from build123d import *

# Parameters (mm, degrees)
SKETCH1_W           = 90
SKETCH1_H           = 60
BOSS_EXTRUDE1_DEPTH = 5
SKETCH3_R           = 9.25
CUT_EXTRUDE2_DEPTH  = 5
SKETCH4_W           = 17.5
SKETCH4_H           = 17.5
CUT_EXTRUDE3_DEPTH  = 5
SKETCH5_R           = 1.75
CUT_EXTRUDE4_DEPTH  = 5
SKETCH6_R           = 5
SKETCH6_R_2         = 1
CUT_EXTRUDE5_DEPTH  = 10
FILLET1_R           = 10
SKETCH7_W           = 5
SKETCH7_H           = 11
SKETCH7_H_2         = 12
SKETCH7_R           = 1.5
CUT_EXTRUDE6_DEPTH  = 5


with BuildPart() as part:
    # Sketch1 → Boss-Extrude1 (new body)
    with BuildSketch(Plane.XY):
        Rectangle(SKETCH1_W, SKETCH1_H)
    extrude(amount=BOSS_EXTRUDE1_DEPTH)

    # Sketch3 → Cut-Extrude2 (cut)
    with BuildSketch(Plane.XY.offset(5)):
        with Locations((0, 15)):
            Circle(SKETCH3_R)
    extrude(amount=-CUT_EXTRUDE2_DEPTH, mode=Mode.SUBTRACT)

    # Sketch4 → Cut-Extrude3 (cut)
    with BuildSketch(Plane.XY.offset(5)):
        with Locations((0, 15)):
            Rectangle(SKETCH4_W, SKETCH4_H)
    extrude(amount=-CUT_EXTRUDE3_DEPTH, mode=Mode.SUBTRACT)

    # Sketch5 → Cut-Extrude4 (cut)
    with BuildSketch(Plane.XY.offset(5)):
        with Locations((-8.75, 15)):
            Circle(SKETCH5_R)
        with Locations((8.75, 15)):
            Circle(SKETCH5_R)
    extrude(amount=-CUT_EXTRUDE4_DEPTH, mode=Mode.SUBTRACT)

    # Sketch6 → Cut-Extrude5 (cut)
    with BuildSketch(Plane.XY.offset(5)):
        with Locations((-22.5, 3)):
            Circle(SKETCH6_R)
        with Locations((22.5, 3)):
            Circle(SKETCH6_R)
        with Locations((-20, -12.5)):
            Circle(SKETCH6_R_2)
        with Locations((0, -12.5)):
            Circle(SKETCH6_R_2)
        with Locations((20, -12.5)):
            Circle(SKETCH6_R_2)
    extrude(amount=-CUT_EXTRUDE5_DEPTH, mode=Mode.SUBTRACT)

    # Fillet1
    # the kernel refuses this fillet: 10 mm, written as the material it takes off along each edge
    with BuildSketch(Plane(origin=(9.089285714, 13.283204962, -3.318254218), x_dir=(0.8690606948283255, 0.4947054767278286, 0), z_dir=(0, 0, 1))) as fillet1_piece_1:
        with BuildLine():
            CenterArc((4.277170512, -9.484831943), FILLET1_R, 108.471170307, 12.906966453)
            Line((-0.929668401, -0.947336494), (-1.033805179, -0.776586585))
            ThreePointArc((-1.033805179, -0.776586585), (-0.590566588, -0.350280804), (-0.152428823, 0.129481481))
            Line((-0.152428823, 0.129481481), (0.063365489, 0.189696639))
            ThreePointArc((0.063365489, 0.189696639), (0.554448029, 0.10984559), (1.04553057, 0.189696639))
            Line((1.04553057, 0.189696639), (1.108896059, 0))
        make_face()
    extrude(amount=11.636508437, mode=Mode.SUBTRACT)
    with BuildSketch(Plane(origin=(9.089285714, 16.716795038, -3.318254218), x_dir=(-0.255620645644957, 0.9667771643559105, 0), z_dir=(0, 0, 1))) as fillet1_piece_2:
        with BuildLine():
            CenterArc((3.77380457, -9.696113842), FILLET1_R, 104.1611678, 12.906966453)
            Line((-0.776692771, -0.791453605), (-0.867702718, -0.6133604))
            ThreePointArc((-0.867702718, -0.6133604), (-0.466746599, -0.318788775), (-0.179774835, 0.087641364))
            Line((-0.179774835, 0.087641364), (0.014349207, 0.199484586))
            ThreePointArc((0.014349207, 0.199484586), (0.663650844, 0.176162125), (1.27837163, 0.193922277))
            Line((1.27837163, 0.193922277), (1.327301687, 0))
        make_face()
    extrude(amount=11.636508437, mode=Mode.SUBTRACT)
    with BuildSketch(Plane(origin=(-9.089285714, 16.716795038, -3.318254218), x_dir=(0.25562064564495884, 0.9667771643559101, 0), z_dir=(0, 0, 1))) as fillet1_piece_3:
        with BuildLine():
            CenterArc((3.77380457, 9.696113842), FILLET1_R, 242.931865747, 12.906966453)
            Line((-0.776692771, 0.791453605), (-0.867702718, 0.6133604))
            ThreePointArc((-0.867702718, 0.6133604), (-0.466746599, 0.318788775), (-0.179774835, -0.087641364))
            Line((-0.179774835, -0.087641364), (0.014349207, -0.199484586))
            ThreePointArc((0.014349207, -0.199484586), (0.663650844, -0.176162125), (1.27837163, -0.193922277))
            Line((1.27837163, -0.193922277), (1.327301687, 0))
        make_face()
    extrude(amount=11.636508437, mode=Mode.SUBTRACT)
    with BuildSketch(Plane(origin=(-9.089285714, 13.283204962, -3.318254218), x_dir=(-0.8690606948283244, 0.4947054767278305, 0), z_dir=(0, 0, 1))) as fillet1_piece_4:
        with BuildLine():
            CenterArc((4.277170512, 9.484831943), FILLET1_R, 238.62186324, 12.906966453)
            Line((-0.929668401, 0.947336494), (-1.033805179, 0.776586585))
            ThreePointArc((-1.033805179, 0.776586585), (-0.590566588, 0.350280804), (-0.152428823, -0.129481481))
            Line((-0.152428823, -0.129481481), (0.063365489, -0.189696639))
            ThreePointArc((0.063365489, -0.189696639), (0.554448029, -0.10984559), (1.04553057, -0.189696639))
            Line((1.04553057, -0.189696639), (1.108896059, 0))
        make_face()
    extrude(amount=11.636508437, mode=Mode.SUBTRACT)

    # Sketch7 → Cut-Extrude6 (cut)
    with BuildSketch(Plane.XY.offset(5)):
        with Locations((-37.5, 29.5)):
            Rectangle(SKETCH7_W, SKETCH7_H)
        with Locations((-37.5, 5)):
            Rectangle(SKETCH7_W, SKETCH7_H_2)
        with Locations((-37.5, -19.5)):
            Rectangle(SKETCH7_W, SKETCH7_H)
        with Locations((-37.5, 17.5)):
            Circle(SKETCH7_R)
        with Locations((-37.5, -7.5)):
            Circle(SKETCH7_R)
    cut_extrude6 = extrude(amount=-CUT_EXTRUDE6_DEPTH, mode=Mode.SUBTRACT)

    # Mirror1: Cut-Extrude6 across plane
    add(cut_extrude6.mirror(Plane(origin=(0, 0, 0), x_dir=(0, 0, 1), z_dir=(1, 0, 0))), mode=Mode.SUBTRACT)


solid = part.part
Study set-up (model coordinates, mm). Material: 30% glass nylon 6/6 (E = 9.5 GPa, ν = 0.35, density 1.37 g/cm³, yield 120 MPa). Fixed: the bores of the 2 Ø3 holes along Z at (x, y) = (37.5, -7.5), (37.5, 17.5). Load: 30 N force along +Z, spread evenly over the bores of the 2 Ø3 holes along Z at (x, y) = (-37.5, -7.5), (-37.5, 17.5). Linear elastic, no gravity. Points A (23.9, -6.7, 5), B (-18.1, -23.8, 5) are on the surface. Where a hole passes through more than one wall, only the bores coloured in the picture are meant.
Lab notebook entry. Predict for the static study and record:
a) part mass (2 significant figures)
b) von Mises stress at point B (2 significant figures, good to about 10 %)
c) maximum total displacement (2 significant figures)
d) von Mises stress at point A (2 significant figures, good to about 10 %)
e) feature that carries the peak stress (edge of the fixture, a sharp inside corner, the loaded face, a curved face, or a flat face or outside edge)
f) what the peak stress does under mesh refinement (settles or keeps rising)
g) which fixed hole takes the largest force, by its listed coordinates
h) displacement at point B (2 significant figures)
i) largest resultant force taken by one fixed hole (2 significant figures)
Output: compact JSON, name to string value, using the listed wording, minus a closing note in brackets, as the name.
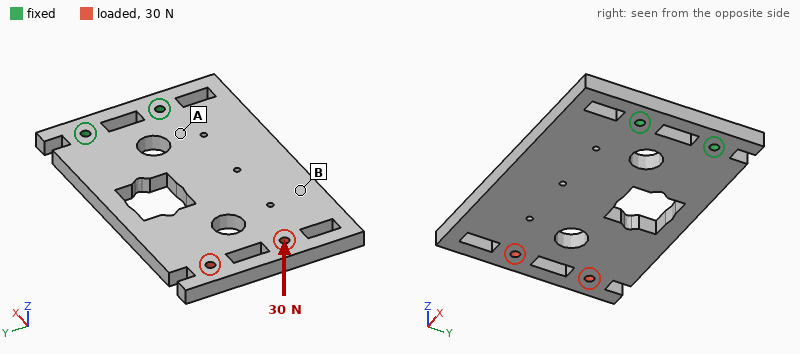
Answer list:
{"part mass": "31 g", "von Mises stress at point B": "3.1 MPa", "maximum total displacement": "1.3 mm", "von Mises stress at point A": "10.0 MPa", "feature that carries the peak stress": "edge of the fixture", "what the peak stress does under mesh refinement": "keeps rising", "which fixed hole takes the largest force, by its listed coordinates": "(37.5, -7.5)", "displacement at point B": "0.67 mm", "largest resultant force taken by one fixed hole": "16 N"}
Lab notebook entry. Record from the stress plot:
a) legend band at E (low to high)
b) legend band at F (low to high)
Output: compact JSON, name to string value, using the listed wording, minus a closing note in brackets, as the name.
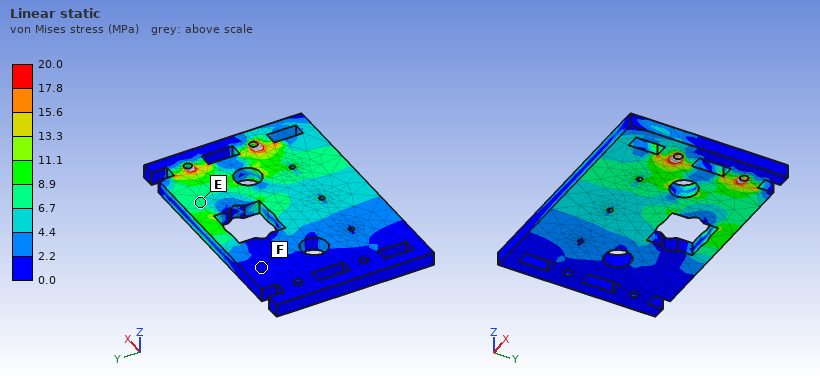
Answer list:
{"legend band at E": "6.7 to 8.9 MPa", "legend band at F": "0.0 to 2.2 MPa"}
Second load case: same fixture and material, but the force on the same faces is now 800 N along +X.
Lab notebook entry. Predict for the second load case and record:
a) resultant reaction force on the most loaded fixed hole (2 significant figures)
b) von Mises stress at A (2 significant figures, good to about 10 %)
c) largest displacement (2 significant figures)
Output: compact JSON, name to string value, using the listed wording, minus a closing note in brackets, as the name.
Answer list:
{"resultant reaction force on the most loaded fixed hole": "400 N", "von Mises stress at A": "5.1 MPa", "largest displacement": "61 µm"}
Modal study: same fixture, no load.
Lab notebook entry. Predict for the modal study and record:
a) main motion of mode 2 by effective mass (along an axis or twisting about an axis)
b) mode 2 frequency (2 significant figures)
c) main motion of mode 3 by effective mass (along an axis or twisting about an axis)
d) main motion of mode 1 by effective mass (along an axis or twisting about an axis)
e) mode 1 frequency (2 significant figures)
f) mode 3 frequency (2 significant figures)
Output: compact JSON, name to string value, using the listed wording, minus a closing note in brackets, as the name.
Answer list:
{"main motion of mode 2 by effective mass": "twisting about X", "mode 2 frequency": "800 Hz", "main motion of mode 3 by effective mass": "along Y", "main motion of mode 1 by effective mass": "along Z", "mode 1 frequency": "270 Hz", "mode 3 frequency": "1600 Hz"}
